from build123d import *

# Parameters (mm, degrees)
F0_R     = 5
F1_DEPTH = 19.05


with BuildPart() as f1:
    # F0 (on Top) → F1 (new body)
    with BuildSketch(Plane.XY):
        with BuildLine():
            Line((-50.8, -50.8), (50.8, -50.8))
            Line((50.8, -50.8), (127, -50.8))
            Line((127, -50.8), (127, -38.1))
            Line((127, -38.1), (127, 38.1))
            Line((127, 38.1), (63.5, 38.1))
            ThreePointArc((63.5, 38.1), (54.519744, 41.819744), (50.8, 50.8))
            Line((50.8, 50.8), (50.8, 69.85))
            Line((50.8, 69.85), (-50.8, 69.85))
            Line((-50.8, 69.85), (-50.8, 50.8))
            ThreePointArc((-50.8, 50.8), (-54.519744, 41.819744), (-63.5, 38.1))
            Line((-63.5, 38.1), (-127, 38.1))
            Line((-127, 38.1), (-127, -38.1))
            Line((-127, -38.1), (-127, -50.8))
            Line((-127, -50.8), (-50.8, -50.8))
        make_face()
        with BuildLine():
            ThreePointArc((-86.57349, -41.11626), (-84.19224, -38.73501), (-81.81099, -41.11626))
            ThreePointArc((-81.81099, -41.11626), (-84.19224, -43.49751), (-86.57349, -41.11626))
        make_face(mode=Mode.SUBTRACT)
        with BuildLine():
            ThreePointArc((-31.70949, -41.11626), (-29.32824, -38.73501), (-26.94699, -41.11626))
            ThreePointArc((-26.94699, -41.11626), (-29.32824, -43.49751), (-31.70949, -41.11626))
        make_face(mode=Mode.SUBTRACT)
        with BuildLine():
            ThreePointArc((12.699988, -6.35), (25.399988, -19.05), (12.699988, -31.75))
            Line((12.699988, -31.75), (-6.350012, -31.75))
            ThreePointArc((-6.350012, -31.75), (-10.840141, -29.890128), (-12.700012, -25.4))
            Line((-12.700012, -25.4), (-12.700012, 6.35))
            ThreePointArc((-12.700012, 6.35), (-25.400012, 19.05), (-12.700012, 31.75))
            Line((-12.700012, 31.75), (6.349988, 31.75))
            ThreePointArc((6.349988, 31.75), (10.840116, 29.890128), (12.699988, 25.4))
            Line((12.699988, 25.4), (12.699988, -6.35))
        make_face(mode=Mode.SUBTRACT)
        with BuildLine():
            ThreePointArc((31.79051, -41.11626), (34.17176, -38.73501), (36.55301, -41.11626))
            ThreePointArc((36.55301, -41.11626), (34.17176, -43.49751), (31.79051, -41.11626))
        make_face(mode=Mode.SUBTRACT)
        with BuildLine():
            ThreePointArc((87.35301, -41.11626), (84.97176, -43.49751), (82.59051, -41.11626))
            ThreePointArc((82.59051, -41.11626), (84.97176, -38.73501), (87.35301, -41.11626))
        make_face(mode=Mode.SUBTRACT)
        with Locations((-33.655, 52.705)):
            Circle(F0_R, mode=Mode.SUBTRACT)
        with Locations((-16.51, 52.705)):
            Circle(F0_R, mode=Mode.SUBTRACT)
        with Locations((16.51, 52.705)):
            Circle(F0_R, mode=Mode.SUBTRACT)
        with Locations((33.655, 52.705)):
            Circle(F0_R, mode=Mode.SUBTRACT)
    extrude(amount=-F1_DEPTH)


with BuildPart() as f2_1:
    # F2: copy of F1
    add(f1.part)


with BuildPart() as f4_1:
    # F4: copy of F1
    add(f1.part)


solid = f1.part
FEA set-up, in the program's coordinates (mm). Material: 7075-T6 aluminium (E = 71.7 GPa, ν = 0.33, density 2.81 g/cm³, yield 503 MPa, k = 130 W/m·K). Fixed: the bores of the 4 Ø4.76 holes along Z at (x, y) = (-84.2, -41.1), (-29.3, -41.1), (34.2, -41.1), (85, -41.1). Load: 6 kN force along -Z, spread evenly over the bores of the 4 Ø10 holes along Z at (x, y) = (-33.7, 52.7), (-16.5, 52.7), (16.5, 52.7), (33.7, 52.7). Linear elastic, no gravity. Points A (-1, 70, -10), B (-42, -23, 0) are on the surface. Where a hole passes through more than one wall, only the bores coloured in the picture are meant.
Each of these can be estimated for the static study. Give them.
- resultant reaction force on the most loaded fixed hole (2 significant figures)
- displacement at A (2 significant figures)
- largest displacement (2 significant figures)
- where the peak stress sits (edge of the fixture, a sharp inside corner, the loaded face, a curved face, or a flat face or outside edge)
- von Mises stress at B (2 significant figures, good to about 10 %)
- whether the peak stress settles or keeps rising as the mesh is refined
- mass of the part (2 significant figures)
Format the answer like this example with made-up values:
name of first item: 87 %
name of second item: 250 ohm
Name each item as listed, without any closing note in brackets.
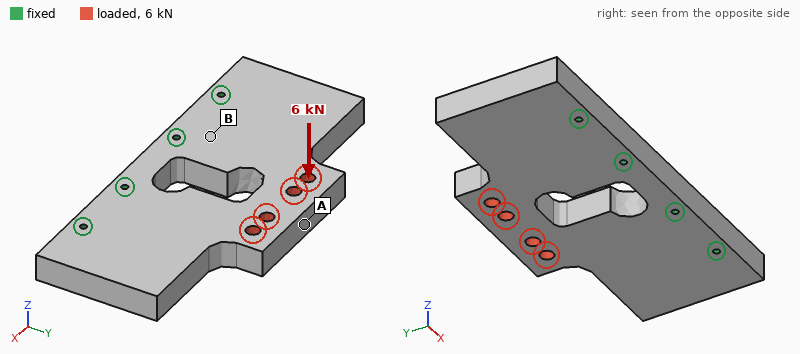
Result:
resultant reaction force on the most loaded fixed hole: 2.5 kN
displacement at A: 0.46 mm
largest displacement: 0.46 mm
where the peak stress sits: edge of the fixture
von Mises stress at B: 37 MPa
whether the peak stress settles or keeps rising as the mesh is refined: keeps rising
mass of the part: 1.3 kg
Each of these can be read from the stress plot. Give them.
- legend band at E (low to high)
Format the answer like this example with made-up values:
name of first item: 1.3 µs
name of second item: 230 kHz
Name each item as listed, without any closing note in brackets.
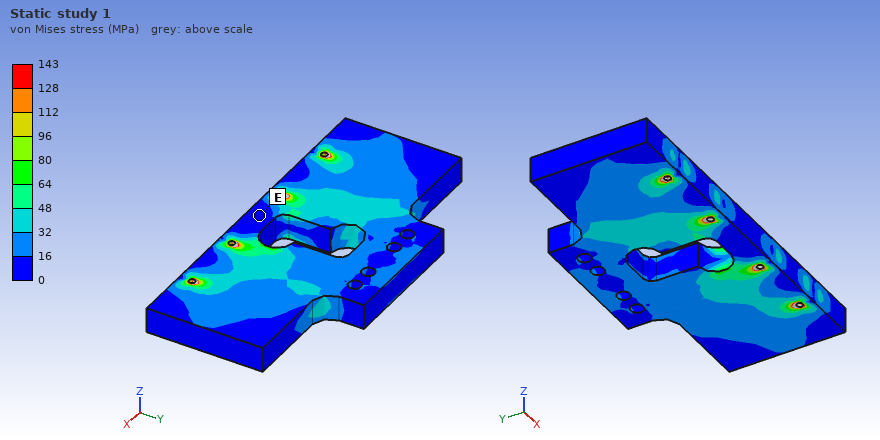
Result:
legend band at E: 0 to 16 MPa
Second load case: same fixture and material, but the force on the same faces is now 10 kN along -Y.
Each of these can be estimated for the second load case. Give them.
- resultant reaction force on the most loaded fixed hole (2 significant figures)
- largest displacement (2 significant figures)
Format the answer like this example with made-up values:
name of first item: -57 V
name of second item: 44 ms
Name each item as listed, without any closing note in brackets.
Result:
resultant reaction force on the most loaded fixed hole: 3.2 kN
largest displacement: 12 µm
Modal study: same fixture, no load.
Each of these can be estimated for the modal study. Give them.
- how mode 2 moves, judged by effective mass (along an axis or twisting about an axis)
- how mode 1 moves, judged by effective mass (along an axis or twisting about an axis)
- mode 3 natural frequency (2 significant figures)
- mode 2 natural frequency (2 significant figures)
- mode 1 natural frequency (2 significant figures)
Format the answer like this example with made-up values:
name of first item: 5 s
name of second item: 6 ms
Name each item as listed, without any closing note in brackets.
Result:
how mode 2 moves, judged by effective mass: twisting about Y
how mode 1 moves, judged by effective mass: along Z
mode 3 natural frequency: 2800 Hz
mode 2 natural frequency: 2000 Hz
mode 1 natural frequency: 1200 Hz
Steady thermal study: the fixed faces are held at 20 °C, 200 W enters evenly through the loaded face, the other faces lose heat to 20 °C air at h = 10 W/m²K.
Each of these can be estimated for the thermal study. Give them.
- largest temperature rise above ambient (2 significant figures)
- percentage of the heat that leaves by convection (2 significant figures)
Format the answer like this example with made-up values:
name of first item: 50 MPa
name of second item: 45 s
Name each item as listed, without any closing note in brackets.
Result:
largest temperature rise above ambient: 73 K
percentage of the heat that leaves by convection: 7.5 %
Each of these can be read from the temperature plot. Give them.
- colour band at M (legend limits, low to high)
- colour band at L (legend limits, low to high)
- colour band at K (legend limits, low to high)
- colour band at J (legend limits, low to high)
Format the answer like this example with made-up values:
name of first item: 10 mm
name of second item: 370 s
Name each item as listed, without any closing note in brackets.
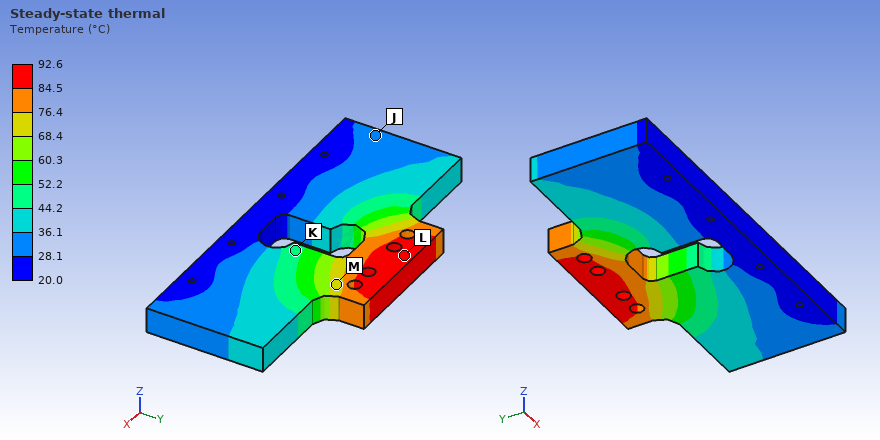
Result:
colour band at M: 68.4 to 76.4 °C
colour band at L: 84.5 to 92.6 °C
colour band at K: 44.2 to 52.2 °C
colour band at J: 28.1 to 36.1 °C
